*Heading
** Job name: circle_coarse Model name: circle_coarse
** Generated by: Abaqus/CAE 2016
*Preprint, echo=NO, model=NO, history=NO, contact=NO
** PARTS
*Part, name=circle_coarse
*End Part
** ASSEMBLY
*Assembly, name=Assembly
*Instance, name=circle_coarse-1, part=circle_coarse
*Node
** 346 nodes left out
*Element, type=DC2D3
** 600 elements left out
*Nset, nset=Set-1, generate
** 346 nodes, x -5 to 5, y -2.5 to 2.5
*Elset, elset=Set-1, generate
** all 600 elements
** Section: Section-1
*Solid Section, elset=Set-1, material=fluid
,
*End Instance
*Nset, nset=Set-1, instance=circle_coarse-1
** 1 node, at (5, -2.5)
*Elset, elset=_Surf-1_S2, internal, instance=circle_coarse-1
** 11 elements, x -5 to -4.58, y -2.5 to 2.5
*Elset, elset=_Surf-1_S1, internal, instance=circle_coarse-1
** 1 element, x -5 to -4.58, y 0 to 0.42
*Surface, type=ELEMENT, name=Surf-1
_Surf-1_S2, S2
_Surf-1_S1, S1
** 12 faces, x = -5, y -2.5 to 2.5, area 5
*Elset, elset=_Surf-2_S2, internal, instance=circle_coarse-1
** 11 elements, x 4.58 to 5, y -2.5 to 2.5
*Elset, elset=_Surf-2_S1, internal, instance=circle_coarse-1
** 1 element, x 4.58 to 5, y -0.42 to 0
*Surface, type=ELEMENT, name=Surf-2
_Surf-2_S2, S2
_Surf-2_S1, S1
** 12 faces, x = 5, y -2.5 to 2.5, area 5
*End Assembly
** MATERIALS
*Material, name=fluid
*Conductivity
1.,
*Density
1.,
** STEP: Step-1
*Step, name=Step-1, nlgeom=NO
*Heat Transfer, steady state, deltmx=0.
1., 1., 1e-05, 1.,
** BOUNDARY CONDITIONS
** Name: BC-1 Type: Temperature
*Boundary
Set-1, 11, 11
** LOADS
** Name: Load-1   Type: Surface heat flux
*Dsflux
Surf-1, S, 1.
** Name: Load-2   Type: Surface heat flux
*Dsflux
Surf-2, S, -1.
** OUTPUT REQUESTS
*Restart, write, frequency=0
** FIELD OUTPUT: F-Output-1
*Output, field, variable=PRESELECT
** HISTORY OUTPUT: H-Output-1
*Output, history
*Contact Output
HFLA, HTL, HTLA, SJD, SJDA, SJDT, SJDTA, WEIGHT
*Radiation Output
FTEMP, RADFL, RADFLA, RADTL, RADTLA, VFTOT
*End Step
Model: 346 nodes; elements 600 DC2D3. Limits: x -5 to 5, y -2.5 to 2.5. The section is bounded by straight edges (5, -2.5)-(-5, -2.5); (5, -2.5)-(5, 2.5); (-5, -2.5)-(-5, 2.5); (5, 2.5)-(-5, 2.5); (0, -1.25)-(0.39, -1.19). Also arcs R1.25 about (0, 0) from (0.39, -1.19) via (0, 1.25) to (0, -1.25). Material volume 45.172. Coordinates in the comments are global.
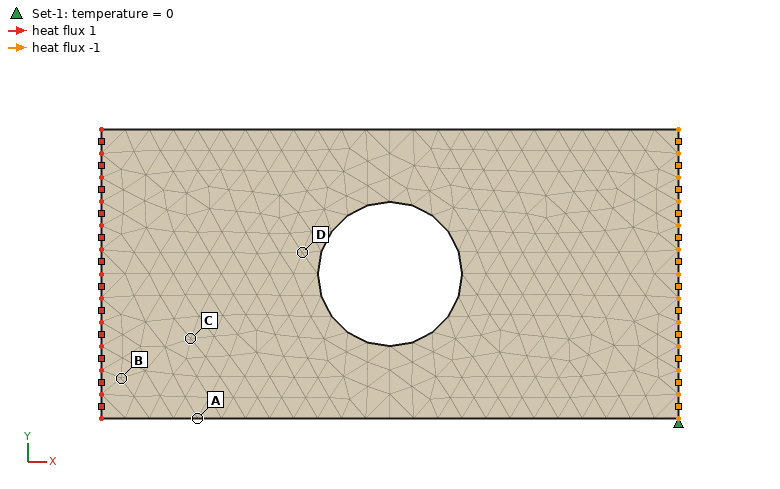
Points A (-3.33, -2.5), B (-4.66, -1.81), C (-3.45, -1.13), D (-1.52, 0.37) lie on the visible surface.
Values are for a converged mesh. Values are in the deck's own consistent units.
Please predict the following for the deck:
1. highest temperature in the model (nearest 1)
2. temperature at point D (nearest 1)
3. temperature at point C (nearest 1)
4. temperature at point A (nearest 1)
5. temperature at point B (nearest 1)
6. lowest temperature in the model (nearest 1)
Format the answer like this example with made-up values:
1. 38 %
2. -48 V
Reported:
1. 12
2. 9
3. 11
4. 11
5. 12
6. 0
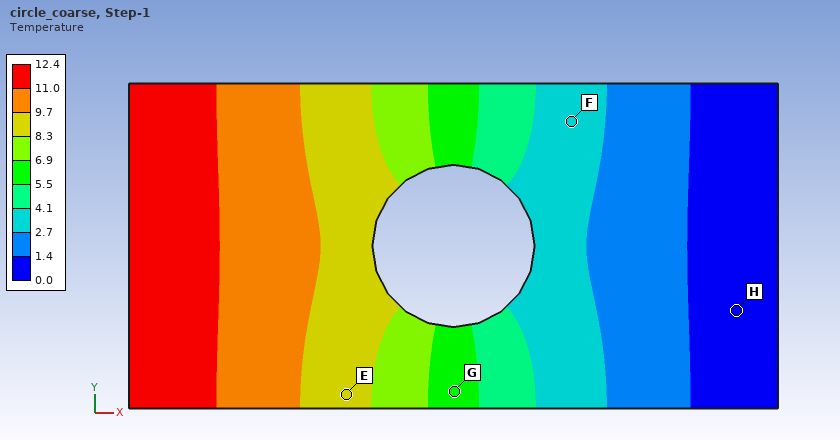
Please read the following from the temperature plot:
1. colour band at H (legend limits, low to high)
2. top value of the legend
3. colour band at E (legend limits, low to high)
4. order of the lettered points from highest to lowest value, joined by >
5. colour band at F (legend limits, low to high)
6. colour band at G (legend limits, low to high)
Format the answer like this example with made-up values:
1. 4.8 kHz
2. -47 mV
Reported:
1. 0.0 to 1.4
2. 12.4
3. 8.3 to 9.7
4. E > G > F > H
5. 2.7 to 4.1
6. 5.5 to 6.9
